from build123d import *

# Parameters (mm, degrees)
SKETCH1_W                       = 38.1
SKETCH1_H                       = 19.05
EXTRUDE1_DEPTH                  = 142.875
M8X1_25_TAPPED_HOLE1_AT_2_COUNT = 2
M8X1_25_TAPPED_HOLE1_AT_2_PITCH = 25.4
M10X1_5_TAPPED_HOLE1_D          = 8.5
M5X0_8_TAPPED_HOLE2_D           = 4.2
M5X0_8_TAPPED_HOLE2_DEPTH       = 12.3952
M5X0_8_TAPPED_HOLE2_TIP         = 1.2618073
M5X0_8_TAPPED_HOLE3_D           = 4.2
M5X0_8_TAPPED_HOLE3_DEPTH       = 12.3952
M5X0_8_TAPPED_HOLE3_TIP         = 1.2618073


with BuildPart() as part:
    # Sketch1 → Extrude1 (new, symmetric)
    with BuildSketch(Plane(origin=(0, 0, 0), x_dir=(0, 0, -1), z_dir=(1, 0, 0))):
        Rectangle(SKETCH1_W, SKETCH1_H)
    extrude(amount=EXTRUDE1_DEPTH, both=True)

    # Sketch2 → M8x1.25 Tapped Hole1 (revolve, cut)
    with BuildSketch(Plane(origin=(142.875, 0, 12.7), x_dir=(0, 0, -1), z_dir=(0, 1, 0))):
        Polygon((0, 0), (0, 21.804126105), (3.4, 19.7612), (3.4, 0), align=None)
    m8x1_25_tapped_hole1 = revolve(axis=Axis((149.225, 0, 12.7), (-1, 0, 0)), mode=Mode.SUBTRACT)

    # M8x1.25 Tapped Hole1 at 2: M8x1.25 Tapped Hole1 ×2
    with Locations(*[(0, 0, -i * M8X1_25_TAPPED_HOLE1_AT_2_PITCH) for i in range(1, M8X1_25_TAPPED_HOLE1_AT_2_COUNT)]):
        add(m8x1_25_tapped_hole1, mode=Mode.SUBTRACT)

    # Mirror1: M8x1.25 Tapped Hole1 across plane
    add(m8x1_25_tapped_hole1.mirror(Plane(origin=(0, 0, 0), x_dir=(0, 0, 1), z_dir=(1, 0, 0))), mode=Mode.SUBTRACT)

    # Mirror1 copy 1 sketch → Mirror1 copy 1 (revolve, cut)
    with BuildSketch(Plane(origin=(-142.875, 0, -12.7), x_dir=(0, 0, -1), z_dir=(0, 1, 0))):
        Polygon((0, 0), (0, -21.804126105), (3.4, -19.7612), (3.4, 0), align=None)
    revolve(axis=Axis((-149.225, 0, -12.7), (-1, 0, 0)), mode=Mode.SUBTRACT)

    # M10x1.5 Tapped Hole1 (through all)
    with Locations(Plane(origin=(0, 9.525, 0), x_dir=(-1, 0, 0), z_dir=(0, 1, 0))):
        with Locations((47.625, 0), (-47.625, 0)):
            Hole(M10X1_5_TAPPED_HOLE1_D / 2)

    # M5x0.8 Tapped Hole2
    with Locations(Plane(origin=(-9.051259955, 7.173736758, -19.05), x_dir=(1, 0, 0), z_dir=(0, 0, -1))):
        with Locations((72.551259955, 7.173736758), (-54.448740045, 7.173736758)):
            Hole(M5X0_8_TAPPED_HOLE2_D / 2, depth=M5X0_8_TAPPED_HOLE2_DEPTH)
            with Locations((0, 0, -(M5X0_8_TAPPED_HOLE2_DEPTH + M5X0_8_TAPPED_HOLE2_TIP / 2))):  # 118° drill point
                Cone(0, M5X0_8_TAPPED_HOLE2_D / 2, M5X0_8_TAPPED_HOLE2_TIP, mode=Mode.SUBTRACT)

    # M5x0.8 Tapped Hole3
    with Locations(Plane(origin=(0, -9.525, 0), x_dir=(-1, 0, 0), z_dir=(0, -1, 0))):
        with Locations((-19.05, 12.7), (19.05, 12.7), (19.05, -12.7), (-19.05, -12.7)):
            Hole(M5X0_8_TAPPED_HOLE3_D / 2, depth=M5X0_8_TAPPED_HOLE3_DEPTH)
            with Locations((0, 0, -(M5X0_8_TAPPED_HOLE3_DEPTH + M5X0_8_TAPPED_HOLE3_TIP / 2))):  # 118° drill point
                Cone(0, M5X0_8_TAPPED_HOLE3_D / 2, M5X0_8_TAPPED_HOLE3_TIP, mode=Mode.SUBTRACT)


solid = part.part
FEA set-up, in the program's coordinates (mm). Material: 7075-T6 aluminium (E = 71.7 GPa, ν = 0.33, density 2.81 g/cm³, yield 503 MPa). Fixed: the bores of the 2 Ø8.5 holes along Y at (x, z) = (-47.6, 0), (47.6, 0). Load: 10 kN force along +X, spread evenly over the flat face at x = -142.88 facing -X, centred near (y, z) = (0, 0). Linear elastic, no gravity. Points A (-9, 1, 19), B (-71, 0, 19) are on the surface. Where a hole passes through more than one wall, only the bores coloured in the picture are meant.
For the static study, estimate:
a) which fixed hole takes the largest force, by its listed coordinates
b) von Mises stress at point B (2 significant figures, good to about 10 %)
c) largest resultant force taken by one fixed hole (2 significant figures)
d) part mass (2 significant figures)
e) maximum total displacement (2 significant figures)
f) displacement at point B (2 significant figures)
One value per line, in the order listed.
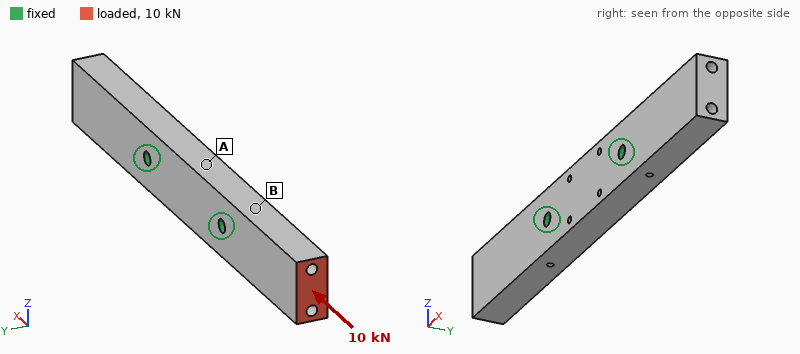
(-47.6, 0)
12 MPa
9.3 kN
570 g
20 µm
5.9 µm
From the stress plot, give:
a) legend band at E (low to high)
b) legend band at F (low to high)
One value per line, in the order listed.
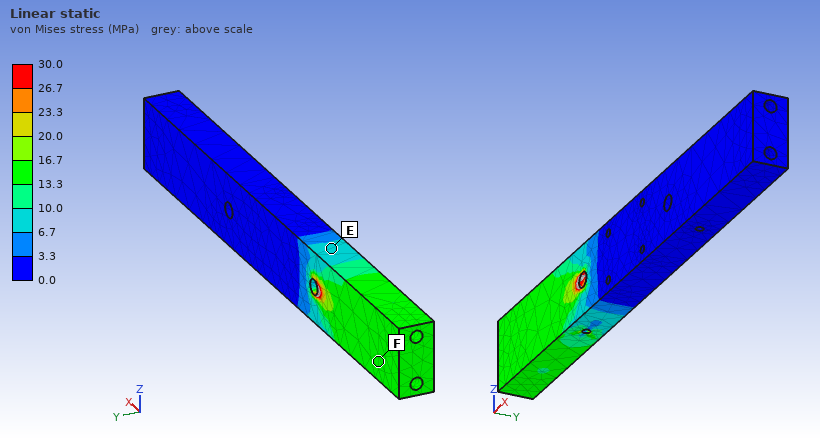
6.7 to 10.0 MPa
13.3 to 16.7 MPa
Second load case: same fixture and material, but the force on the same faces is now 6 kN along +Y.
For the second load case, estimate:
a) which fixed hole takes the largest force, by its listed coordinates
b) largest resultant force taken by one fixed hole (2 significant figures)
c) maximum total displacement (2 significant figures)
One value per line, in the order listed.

(-47.6, 0)
7.0 kN
1.2 mm
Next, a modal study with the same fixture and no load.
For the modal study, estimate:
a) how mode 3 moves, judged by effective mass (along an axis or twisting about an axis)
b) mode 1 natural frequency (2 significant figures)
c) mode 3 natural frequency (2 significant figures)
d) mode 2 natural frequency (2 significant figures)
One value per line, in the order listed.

along Z
1700 Hz
2300 Hz
1700 Hz
